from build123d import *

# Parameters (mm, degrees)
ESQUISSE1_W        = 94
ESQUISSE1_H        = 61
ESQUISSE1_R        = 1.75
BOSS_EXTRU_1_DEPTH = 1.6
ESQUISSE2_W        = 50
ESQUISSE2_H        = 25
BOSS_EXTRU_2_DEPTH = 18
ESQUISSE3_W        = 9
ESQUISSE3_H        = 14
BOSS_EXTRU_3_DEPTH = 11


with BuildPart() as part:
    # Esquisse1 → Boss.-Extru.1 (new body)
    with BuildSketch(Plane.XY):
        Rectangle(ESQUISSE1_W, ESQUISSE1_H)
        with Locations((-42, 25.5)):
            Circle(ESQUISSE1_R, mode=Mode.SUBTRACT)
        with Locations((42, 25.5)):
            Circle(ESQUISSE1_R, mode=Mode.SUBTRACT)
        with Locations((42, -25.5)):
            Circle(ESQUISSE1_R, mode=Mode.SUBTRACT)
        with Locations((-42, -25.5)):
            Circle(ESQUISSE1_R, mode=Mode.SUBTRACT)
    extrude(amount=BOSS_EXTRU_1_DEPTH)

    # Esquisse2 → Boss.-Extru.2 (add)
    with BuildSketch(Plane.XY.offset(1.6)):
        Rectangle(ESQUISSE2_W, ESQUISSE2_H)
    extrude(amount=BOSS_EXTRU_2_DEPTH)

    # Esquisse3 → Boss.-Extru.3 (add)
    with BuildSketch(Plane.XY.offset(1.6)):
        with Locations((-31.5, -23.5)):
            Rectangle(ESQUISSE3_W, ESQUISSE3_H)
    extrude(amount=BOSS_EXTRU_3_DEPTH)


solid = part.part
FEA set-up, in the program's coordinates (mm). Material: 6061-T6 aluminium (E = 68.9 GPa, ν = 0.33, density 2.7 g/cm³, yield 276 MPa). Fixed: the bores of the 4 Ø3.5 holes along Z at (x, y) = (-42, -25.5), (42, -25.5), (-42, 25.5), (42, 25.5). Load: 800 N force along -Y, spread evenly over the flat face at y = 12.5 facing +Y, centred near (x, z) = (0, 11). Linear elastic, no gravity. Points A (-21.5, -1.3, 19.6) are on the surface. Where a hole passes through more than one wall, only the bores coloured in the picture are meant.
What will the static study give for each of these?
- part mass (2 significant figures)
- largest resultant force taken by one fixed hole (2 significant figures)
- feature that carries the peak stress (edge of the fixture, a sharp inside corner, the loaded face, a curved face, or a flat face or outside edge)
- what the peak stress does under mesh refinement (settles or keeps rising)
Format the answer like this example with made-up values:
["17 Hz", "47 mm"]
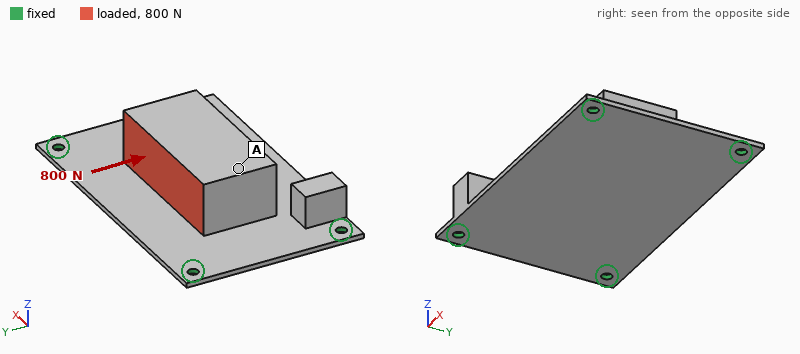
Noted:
["89 g", "270 N", "edge of the fixture", "keeps rising"]
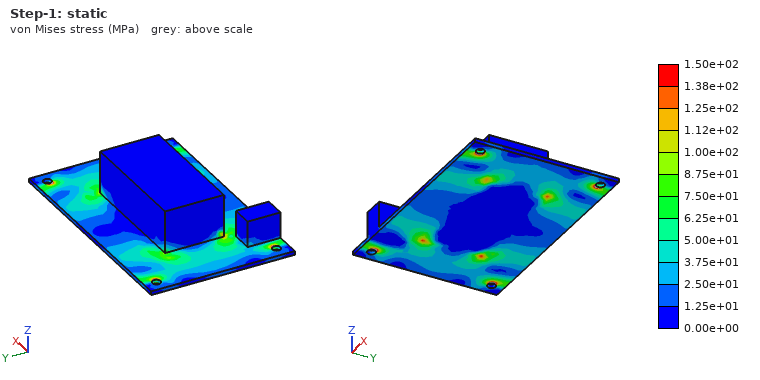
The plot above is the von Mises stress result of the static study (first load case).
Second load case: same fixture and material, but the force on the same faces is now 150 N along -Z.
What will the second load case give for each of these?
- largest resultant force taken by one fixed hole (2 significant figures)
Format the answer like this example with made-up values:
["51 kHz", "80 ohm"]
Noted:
["61 N"]
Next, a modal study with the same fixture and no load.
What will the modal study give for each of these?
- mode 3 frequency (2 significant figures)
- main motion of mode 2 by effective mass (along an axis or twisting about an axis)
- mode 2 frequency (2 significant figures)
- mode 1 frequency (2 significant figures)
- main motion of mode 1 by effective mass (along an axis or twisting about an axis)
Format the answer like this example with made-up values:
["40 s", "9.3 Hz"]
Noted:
["1600 Hz", "along Y", "1200 Hz", "820 Hz", "along Z"]
